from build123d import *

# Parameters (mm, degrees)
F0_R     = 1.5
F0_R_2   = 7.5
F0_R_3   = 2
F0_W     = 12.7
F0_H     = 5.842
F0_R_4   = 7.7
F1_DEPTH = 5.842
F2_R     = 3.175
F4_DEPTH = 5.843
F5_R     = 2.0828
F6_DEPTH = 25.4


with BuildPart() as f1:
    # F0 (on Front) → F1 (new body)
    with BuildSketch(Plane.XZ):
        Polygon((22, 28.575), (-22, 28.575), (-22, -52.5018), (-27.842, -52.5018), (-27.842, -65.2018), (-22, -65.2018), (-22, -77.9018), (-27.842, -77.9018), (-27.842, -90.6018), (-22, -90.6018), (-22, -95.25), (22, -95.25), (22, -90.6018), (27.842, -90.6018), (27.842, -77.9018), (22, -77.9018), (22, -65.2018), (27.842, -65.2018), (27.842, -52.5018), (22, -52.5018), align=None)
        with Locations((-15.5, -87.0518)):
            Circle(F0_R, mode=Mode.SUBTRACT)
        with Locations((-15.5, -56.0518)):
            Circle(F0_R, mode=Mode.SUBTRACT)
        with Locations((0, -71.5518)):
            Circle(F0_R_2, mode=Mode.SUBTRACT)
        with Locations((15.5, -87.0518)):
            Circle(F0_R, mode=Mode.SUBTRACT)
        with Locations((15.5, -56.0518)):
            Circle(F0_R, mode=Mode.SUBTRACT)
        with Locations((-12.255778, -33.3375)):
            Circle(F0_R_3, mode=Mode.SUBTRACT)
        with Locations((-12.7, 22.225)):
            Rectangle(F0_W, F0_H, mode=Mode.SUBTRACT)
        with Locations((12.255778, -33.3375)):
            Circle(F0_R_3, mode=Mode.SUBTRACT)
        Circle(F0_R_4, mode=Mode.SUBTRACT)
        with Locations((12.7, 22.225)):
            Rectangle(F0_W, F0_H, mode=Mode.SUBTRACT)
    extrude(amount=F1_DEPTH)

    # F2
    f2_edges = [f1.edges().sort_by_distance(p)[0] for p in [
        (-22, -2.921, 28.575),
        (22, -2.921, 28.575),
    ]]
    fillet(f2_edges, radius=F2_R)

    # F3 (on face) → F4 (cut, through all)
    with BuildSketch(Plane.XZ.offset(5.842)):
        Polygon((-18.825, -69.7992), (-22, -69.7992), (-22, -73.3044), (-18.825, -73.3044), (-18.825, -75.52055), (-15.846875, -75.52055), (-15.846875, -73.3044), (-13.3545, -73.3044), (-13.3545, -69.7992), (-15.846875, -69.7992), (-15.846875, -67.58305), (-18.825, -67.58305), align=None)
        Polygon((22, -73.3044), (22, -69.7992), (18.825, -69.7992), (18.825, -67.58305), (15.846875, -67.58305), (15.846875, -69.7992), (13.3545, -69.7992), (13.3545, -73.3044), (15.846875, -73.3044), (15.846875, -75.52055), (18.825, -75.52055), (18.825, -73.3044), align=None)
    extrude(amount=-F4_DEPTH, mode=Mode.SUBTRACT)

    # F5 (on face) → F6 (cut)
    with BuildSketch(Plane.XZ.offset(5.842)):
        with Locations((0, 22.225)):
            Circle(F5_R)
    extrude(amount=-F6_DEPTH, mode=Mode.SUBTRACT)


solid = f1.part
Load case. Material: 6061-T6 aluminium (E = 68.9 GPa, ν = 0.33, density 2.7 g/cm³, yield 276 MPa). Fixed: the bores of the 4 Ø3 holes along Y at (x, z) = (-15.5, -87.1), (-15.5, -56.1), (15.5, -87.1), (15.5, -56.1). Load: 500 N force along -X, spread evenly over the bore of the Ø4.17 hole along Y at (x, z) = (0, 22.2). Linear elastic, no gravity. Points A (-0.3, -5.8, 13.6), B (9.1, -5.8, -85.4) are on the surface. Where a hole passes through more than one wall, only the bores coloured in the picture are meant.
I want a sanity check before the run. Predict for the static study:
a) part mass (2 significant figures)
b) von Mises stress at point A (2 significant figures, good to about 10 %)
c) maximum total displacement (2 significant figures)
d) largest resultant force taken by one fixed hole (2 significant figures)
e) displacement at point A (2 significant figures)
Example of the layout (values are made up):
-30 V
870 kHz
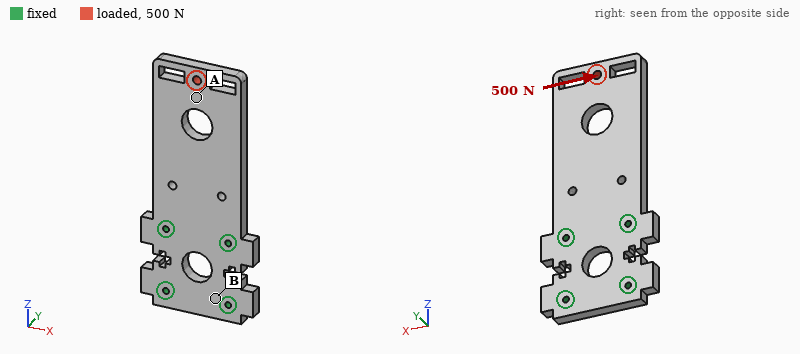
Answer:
80 g
6.9 MPa
48 µm
1.2 kN
35 µm
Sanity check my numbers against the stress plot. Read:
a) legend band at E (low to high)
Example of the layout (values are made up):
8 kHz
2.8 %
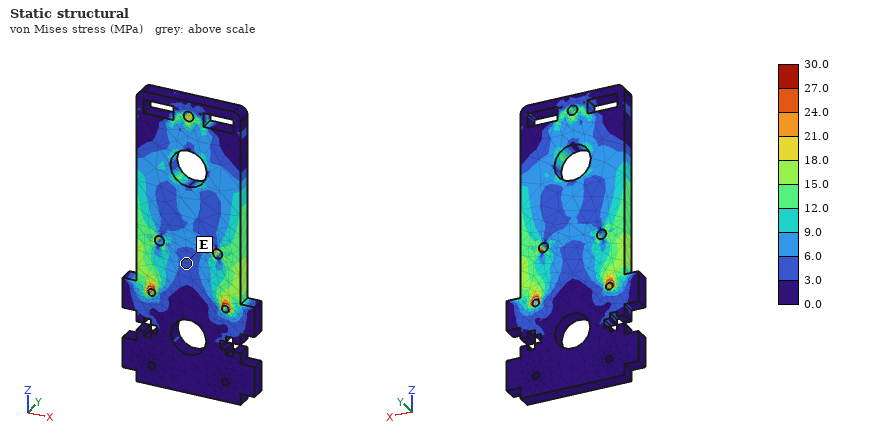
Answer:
3.0 to 6.0 MPa
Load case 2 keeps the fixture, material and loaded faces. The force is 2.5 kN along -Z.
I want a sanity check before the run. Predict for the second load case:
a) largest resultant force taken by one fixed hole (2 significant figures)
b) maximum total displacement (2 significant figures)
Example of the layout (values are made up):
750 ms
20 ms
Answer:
1.1 kN
25 µm
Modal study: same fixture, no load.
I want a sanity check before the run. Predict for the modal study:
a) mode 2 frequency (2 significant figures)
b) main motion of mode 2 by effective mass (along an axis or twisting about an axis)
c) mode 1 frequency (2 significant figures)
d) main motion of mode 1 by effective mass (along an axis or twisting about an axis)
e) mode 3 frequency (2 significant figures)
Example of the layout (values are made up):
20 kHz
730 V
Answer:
2700 Hz
twisting about Z
700 Hz
along Y
3900 Hz
